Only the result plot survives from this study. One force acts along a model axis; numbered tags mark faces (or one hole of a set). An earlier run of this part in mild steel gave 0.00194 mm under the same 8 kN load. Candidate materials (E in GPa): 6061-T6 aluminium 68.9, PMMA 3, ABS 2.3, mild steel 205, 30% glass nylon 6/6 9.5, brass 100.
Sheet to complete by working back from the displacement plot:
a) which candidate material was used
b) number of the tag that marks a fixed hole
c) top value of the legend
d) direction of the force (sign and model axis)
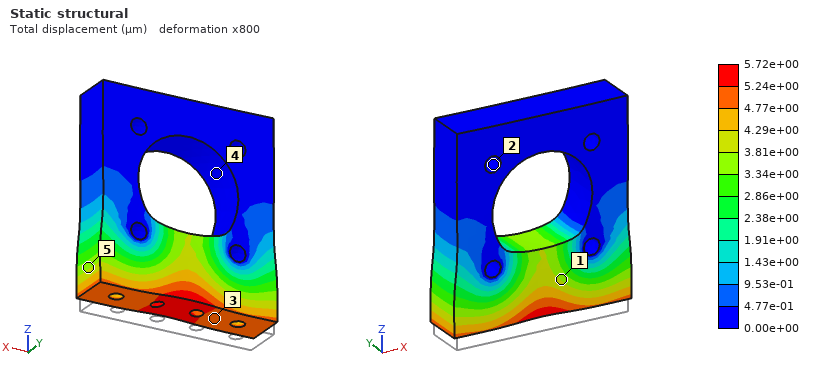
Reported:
6061-T6 aluminium
2
5.72e+00 µm
+Z
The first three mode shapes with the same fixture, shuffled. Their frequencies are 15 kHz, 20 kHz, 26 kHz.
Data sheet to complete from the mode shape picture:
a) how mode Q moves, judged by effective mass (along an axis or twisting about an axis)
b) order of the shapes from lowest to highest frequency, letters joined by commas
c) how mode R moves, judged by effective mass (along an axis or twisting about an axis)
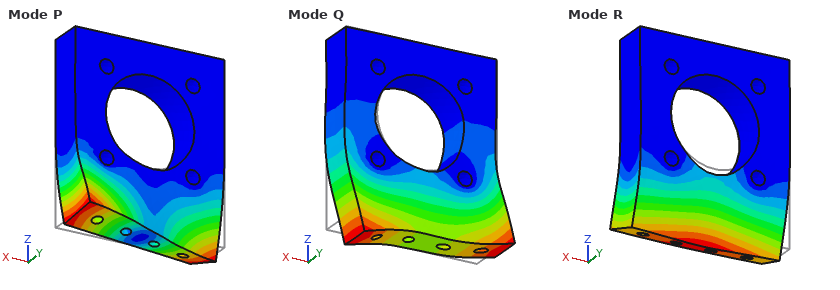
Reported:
along X
R, P, Q
along Y
